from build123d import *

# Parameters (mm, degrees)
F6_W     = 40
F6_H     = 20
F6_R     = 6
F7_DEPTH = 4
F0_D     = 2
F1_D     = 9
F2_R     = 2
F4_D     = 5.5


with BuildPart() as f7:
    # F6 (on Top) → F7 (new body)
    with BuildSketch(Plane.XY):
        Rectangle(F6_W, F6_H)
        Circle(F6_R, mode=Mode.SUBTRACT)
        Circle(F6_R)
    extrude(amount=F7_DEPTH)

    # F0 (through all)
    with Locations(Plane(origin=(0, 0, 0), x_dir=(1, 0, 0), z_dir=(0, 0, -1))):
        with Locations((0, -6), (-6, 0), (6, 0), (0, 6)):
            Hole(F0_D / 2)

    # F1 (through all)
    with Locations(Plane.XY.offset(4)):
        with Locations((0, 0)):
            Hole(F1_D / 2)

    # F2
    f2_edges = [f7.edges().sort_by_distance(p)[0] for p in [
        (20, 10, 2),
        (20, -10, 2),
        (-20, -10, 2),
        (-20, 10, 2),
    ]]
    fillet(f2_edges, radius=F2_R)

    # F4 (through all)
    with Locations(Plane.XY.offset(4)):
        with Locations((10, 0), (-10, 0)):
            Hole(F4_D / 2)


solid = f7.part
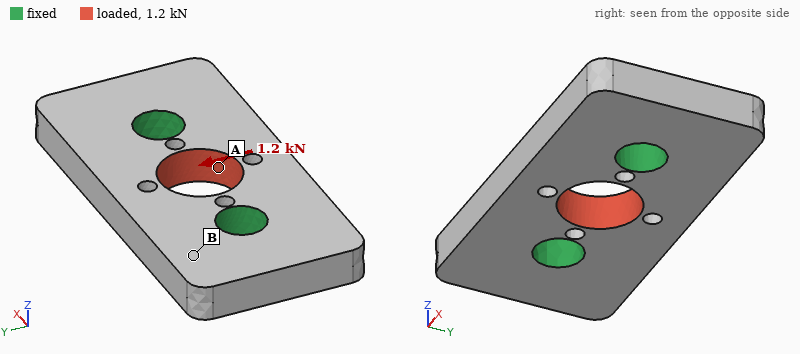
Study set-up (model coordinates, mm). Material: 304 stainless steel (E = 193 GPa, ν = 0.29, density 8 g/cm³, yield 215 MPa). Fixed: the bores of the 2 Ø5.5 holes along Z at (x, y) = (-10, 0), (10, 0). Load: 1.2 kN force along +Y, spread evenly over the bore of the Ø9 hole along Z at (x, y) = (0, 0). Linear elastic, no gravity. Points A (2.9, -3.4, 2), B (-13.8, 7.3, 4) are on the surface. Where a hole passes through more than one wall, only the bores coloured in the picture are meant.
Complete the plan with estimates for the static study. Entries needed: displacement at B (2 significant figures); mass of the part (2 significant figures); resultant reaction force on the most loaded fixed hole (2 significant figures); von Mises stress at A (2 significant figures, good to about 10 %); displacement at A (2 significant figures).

0.24 µm
22 g
600 N
18 MPa
1.0 µm
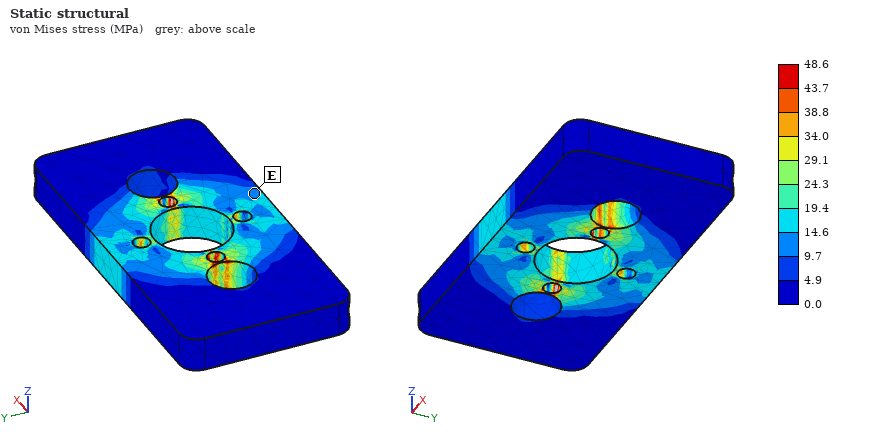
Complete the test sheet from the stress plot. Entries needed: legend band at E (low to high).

9.7 to 14.6 MPa
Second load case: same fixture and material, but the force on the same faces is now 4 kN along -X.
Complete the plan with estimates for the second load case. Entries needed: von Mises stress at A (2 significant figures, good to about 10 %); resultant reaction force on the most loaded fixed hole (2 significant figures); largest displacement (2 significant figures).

62 MPa
2.0 kN
2.1 µm
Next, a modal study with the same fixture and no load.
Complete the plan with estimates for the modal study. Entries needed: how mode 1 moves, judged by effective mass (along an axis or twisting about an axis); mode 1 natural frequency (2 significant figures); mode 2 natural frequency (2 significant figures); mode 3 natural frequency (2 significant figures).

twisting about X
30 kHz
31 kHz
31 kHz
